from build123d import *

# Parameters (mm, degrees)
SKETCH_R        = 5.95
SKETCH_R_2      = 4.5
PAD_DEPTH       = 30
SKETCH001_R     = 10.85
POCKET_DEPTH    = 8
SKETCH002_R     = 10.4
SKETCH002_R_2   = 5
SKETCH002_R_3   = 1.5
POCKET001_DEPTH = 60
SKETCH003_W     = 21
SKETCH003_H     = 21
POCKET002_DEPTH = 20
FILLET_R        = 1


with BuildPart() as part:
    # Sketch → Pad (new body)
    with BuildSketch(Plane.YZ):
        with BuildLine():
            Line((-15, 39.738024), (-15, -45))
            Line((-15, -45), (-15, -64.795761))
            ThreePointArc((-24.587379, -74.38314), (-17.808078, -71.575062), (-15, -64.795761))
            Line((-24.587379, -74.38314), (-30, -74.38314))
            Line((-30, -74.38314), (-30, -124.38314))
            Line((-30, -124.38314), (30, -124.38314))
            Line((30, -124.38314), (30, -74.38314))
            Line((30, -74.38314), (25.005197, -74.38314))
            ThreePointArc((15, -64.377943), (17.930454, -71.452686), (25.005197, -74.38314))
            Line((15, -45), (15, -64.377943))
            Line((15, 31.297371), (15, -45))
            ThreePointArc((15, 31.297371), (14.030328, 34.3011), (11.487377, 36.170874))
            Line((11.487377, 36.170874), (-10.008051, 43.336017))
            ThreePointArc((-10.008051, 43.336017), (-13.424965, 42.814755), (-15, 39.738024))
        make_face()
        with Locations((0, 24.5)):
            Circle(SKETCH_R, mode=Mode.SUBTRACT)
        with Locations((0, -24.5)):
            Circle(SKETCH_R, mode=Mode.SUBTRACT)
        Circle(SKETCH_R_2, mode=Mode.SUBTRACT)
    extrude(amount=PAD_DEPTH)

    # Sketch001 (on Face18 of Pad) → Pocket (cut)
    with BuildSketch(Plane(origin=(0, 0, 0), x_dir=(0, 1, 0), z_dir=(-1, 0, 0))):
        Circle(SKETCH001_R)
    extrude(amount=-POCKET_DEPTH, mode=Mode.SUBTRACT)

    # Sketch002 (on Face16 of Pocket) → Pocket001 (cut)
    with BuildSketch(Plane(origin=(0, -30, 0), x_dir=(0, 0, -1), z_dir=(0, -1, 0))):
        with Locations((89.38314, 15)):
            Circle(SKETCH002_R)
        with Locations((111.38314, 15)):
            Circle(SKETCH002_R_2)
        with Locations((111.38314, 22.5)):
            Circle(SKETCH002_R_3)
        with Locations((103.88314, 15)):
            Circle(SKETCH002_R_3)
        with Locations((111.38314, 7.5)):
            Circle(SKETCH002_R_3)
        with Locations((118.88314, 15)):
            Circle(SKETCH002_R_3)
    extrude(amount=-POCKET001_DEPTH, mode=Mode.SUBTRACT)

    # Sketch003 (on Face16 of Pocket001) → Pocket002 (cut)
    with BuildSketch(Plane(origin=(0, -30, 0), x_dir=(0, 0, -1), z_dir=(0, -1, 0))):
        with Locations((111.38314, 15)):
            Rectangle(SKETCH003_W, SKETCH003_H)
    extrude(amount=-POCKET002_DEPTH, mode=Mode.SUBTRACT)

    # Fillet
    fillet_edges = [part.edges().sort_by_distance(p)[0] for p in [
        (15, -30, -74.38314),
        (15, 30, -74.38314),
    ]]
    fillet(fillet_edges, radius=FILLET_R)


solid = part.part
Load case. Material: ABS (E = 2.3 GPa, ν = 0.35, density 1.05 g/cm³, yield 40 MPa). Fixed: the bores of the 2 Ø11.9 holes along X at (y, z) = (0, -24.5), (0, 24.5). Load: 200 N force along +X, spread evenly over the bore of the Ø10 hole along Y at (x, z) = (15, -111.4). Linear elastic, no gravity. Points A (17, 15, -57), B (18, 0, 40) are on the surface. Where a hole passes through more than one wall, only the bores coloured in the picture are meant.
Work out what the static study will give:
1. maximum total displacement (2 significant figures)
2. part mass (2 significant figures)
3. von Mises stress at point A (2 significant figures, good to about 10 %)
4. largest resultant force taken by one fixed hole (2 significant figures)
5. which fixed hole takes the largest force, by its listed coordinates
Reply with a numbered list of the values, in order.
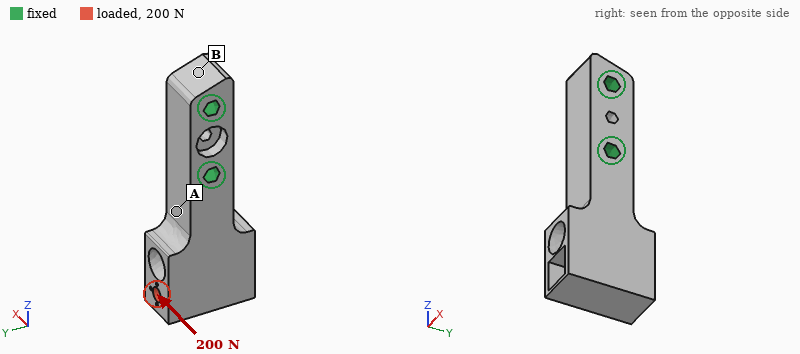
1. 0.43 mm
2. 160 g
3. 1.3 MPa
4. 230 N
5. (0, -24.5)
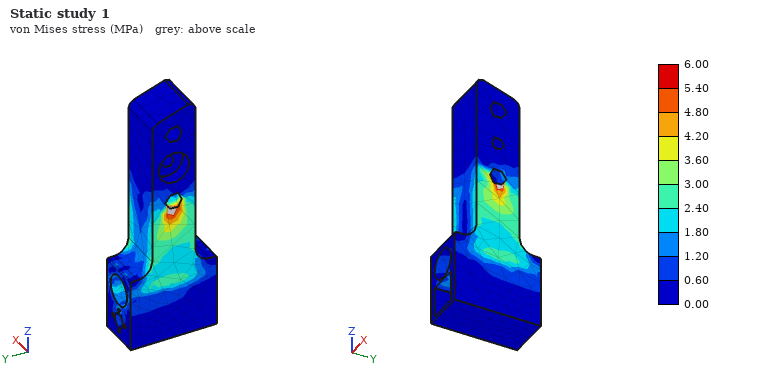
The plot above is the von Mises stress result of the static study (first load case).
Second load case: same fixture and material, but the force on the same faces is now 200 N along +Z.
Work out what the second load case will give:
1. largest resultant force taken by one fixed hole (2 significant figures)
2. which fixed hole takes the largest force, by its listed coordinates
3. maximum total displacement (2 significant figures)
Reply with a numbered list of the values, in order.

1. 190 N
2. (0, -24.5)
3. 75 µm
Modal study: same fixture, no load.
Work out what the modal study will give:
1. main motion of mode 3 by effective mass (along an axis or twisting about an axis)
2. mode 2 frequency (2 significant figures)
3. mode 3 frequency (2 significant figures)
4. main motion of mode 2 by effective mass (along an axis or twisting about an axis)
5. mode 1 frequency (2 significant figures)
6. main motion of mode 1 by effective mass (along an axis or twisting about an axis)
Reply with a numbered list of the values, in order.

1. twisting about Z
2. 590 Hz
3. 1300 Hz
4. along X
5. 530 Hz
6. along Y
